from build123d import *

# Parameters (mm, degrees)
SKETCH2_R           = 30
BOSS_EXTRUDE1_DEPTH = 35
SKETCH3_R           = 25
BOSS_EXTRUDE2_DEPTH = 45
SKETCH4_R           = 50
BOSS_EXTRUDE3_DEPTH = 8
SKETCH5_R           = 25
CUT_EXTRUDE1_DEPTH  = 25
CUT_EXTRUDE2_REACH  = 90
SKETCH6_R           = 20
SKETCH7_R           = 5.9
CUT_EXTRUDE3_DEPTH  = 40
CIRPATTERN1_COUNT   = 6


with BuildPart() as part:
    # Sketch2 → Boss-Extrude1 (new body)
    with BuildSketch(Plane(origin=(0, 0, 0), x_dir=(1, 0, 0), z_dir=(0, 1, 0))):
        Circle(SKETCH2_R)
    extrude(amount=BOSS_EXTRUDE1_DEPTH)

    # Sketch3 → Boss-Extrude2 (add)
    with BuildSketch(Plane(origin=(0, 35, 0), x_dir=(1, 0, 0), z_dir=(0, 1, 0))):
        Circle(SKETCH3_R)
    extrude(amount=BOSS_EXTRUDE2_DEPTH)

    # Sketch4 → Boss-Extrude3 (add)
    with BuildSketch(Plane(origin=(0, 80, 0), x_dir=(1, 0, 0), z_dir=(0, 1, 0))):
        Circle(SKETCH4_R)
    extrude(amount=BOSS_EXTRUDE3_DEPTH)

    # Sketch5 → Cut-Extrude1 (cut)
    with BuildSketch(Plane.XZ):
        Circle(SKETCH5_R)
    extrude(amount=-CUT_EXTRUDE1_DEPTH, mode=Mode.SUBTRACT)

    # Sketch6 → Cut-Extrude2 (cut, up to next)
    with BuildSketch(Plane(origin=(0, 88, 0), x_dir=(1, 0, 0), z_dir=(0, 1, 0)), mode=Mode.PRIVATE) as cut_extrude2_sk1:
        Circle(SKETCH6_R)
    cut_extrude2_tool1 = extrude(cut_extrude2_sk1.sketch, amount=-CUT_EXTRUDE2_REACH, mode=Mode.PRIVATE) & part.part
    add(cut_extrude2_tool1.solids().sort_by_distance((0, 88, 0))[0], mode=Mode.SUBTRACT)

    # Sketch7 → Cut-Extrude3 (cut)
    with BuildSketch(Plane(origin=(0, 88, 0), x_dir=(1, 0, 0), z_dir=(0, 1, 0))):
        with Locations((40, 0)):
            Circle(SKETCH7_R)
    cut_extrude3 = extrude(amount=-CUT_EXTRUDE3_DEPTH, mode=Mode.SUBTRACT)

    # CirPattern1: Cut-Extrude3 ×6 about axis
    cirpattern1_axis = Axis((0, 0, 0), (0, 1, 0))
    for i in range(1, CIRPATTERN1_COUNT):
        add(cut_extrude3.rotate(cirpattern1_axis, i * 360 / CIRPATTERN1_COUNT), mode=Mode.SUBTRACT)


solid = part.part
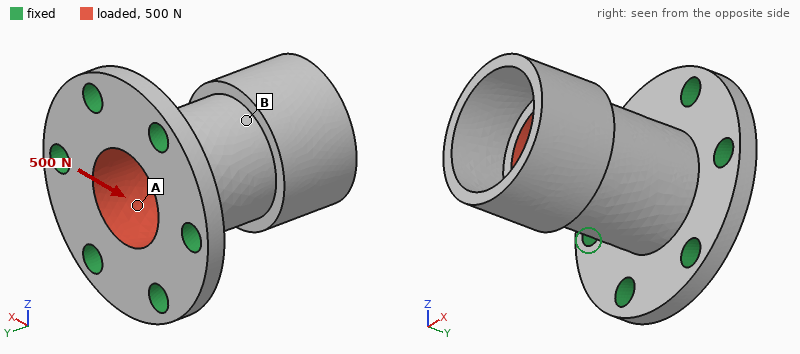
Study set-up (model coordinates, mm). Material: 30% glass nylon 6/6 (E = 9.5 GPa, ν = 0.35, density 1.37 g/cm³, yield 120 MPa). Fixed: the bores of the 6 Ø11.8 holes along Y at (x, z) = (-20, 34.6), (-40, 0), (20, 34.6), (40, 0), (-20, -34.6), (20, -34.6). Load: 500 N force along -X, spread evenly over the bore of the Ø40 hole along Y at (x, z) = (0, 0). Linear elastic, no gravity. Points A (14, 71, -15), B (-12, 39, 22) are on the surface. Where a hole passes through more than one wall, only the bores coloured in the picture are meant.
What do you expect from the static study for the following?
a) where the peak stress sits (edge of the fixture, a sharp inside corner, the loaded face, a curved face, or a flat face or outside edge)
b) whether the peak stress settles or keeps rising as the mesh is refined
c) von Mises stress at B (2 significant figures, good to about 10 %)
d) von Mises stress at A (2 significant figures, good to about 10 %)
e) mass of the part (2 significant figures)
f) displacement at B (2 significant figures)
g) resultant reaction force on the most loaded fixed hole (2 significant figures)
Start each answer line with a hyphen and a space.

- edge of the fixture
- keeps rising
- 0.51 MPa
- 1.4 MPa
- 160 g
- 25 µm
- 190 N
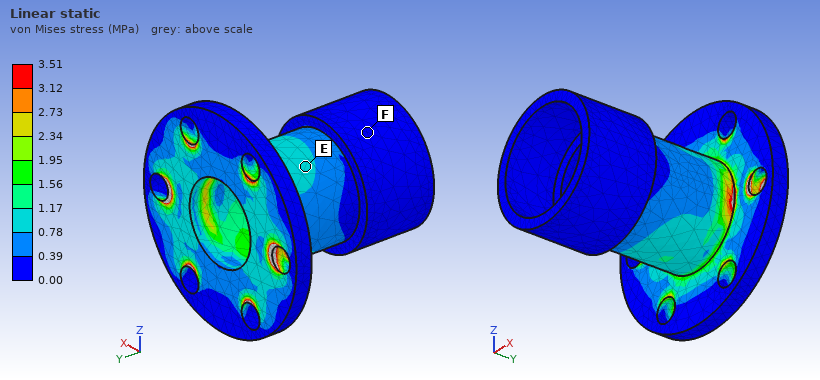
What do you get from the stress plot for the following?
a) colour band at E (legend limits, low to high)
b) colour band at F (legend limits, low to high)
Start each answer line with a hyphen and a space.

- 0.78 to 1.17 MPa
- 0.00 to 0.39 MPa
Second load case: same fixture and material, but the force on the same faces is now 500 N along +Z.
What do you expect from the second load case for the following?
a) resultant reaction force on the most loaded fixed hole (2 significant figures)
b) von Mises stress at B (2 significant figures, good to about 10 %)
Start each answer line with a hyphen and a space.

- 170 N
- 0.36 MPa
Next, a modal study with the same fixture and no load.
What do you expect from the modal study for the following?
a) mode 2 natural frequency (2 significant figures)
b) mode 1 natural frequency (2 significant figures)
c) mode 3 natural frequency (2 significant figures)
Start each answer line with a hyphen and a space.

- 1500 Hz
- 1500 Hz
- 3200 Hz
